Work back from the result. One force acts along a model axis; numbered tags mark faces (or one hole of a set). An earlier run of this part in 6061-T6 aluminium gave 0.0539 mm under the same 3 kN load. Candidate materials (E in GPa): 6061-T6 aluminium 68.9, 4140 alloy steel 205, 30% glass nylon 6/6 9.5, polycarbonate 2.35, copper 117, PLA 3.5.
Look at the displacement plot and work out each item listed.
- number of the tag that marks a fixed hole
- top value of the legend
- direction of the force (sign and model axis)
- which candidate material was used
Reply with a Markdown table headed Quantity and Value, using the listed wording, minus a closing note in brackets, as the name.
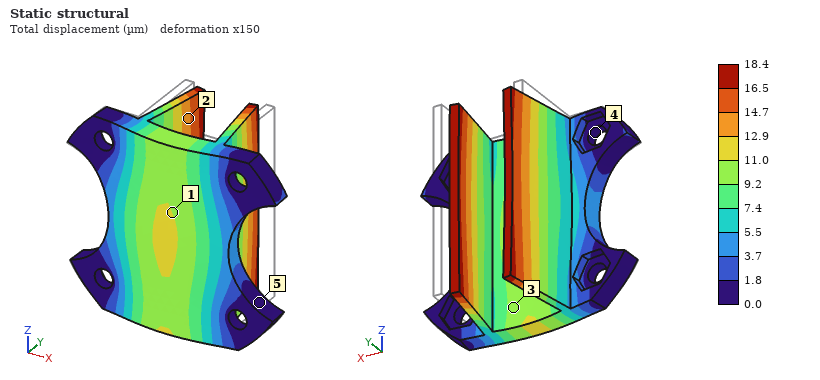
| Quantity | Value |
|---|---|
| number of the tag that marks a fixed hole | 4 |
| top value of the legend | 18.4 µm |
| direction of the force | -Y |
| which candidate material was used | 4140 alloy steel |
